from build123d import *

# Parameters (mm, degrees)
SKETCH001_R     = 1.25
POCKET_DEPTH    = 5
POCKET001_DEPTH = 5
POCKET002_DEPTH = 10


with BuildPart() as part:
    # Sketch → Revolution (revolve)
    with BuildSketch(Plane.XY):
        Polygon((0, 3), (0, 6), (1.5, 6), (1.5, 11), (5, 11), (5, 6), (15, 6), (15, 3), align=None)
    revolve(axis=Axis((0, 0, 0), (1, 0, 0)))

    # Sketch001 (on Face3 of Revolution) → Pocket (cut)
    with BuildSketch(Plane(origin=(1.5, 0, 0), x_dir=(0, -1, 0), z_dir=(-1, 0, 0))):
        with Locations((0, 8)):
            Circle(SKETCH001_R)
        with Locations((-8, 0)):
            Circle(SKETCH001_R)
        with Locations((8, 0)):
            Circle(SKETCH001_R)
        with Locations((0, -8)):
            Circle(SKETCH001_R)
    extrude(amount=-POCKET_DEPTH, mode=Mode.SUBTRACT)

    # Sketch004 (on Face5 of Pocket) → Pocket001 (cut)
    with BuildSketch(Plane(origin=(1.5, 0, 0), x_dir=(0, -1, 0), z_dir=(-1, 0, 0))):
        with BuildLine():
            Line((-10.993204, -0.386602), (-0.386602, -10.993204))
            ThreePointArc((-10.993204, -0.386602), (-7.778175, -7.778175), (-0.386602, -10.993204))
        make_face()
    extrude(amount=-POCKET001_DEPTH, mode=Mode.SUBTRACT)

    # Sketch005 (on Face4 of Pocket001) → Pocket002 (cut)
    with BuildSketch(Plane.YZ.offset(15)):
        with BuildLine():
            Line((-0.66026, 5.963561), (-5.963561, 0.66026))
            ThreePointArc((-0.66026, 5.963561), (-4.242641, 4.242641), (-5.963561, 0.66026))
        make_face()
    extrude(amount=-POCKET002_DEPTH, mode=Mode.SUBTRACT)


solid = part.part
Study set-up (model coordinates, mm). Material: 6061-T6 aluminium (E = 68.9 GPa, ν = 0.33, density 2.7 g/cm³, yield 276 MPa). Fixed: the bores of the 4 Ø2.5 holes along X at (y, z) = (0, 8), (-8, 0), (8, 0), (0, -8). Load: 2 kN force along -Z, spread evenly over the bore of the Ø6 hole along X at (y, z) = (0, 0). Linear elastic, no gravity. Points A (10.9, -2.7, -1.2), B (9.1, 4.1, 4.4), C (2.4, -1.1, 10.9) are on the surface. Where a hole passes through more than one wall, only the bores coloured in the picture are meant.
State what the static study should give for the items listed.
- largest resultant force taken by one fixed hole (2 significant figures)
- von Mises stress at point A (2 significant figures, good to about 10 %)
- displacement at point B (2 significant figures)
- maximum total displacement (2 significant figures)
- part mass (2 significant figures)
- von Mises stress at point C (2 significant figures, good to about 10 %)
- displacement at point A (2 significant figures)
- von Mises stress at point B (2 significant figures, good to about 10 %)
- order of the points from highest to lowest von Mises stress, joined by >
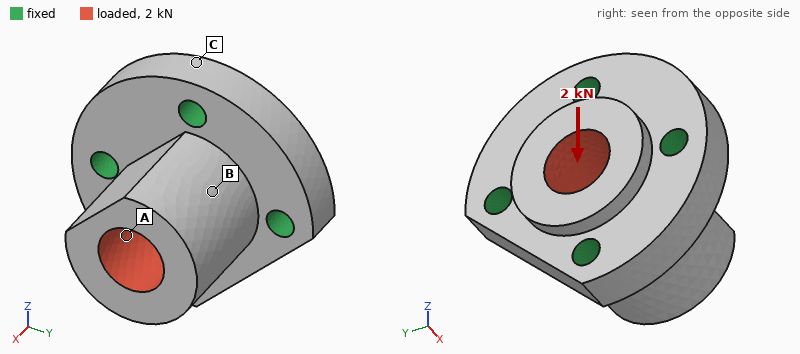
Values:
870 N
33 MPa
8.2 µm
16 µm
5.3 g
9.5 MPa
11 µm
16 MPa
A > B > C
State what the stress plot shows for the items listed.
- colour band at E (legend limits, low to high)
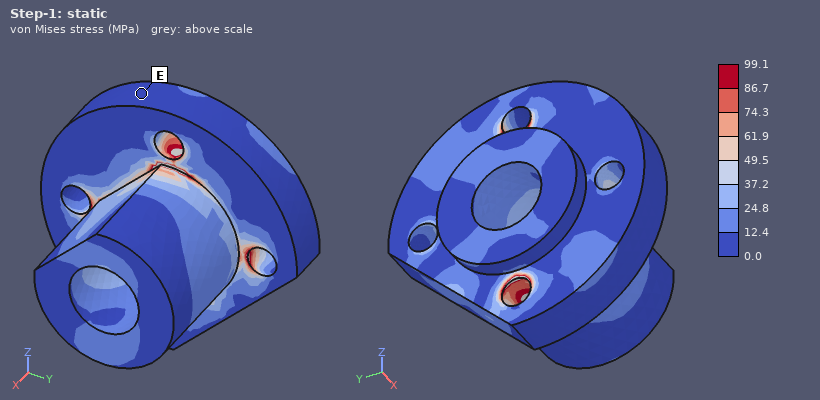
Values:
0.0 to 12.4 MPa
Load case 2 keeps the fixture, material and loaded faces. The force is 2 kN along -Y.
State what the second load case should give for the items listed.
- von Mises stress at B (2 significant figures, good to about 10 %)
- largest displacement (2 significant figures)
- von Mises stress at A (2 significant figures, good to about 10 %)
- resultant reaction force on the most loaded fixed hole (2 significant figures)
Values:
20 MPa
16 µm
23 MPa
870 N
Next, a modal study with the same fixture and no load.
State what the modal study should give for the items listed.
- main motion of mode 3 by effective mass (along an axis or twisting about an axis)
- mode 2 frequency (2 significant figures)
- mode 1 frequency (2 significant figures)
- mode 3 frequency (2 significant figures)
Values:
along X
38 kHz
37 kHz
66 kHz
